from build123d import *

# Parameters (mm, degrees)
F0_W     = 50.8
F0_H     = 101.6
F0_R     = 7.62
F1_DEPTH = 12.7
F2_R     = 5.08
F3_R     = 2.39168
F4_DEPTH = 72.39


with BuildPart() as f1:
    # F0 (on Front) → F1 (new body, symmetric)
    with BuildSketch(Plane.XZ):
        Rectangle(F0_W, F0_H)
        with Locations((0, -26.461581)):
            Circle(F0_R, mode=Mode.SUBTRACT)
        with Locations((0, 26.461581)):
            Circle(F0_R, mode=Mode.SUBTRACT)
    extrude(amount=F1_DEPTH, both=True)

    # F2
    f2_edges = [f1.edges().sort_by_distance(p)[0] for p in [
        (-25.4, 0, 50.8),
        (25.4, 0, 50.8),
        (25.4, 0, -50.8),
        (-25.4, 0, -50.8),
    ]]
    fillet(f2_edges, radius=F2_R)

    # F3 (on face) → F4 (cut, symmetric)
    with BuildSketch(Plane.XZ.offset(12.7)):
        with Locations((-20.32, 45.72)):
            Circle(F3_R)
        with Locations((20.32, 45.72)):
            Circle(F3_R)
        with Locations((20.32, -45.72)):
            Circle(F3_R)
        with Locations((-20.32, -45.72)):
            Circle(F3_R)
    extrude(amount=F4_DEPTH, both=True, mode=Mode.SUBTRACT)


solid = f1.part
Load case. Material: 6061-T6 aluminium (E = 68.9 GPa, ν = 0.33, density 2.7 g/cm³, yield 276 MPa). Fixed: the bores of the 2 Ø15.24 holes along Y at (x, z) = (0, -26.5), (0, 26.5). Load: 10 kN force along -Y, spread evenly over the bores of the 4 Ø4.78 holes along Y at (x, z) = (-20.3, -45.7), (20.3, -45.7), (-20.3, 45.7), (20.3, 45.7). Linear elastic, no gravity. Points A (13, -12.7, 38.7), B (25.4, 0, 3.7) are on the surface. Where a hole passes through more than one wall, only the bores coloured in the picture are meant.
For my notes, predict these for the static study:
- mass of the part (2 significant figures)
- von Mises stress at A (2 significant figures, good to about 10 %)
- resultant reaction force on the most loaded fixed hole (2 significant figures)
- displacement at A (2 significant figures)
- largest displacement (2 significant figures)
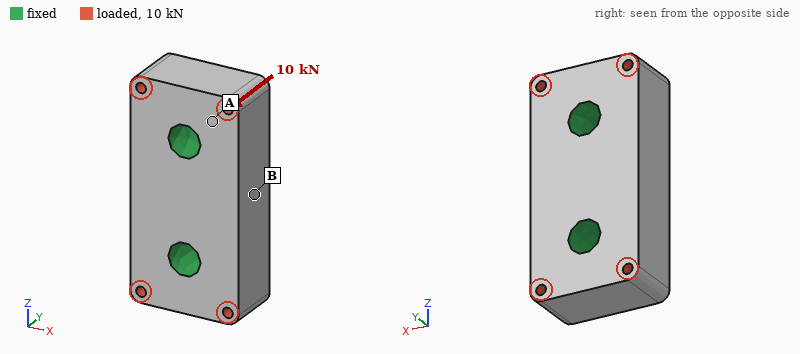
320 g
9.8 MPa
5.0 kN
4.3 µm
10 µm
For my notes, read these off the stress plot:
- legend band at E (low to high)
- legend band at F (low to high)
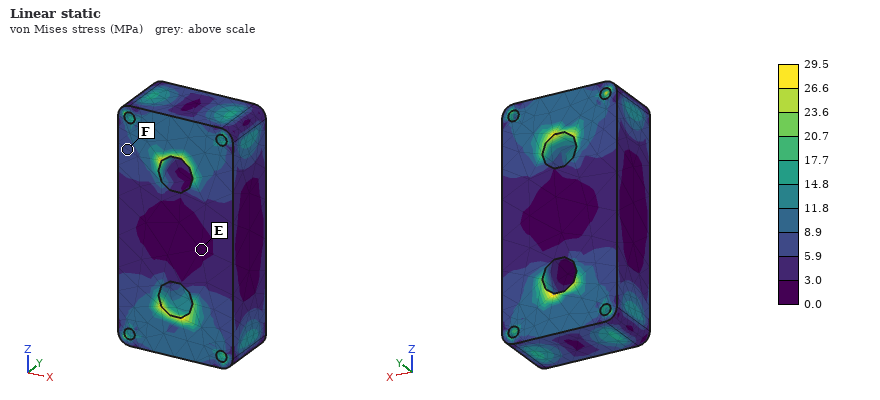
0.0 to 3.0 MPa
5.9 to 8.9 MPa
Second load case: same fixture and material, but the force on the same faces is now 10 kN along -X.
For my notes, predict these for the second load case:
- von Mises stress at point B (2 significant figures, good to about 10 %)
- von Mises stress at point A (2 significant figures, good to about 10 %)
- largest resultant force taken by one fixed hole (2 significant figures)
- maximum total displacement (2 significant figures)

4.4 MPa
8.3 MPa
5.0 kN
7.0 µm
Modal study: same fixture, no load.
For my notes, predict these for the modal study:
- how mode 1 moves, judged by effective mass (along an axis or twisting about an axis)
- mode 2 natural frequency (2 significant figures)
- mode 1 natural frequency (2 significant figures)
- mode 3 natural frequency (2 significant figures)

twisting about Z
22 kHz
20 kHz
23 kHz
